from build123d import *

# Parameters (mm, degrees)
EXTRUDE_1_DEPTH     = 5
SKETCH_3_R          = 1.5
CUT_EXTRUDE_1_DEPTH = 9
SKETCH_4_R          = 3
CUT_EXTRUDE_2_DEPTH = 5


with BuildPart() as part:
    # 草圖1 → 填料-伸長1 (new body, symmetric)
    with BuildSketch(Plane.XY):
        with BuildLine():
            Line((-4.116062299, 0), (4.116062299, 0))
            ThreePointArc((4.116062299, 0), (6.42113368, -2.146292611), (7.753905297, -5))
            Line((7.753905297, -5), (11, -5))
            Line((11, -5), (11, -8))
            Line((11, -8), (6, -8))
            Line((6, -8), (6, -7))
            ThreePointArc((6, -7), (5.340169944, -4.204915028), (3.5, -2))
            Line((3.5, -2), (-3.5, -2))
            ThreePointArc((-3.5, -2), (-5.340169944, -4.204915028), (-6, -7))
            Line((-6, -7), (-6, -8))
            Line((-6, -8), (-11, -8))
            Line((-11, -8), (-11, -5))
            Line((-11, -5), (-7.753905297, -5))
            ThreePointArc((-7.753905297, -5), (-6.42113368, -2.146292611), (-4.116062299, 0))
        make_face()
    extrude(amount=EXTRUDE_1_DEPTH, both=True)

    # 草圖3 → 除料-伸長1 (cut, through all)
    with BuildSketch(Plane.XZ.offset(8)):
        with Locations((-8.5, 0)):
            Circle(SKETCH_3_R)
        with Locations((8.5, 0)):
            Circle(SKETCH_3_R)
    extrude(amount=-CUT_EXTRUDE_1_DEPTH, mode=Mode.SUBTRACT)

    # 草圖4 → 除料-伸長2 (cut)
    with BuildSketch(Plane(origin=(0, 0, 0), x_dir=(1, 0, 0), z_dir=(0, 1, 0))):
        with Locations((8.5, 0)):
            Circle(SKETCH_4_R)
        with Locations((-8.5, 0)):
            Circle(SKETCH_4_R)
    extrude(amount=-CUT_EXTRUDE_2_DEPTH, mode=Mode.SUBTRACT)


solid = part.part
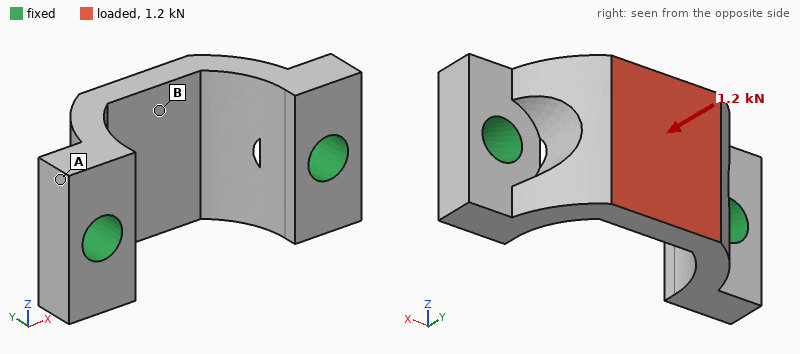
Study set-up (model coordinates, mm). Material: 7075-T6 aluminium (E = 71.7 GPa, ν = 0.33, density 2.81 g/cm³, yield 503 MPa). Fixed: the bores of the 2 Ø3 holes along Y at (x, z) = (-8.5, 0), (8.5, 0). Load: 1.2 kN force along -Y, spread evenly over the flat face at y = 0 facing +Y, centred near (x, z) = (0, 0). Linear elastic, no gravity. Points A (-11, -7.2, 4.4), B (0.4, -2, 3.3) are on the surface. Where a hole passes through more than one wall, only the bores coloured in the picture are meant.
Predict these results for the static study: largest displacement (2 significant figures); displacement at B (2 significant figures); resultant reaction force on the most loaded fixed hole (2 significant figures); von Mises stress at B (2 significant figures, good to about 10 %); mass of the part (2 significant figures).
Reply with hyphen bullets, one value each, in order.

- 25 µm
- 24 µm
- 750 N
- 96 MPa
- 1.6 g
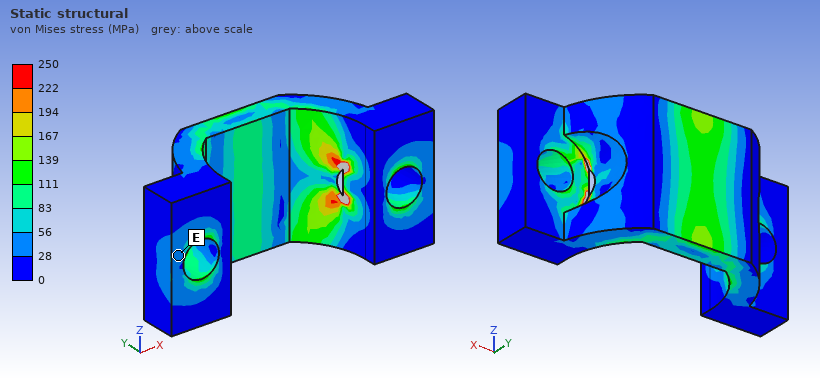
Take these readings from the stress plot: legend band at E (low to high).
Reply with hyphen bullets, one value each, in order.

- 28 to 56 MPa
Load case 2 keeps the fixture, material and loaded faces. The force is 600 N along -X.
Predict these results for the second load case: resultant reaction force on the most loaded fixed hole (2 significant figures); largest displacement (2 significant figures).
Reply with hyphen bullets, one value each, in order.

- 350 N
- 15 µm
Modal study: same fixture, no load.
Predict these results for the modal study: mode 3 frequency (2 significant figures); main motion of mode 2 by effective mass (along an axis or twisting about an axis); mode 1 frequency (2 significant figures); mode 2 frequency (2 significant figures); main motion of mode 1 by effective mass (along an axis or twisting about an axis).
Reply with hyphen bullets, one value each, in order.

- 48 kHz
- along X
- 32 kHz
- 36 kHz
- along Z
